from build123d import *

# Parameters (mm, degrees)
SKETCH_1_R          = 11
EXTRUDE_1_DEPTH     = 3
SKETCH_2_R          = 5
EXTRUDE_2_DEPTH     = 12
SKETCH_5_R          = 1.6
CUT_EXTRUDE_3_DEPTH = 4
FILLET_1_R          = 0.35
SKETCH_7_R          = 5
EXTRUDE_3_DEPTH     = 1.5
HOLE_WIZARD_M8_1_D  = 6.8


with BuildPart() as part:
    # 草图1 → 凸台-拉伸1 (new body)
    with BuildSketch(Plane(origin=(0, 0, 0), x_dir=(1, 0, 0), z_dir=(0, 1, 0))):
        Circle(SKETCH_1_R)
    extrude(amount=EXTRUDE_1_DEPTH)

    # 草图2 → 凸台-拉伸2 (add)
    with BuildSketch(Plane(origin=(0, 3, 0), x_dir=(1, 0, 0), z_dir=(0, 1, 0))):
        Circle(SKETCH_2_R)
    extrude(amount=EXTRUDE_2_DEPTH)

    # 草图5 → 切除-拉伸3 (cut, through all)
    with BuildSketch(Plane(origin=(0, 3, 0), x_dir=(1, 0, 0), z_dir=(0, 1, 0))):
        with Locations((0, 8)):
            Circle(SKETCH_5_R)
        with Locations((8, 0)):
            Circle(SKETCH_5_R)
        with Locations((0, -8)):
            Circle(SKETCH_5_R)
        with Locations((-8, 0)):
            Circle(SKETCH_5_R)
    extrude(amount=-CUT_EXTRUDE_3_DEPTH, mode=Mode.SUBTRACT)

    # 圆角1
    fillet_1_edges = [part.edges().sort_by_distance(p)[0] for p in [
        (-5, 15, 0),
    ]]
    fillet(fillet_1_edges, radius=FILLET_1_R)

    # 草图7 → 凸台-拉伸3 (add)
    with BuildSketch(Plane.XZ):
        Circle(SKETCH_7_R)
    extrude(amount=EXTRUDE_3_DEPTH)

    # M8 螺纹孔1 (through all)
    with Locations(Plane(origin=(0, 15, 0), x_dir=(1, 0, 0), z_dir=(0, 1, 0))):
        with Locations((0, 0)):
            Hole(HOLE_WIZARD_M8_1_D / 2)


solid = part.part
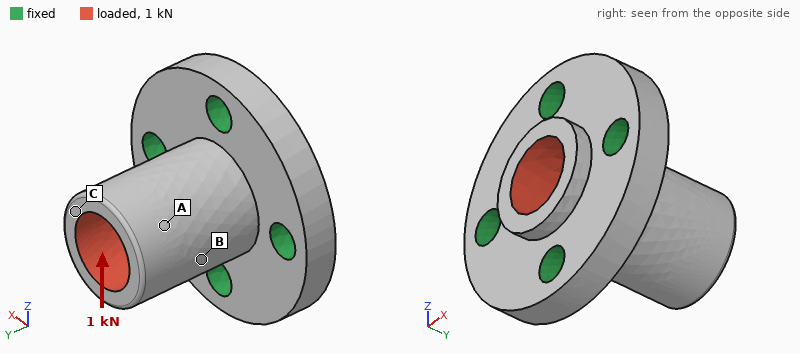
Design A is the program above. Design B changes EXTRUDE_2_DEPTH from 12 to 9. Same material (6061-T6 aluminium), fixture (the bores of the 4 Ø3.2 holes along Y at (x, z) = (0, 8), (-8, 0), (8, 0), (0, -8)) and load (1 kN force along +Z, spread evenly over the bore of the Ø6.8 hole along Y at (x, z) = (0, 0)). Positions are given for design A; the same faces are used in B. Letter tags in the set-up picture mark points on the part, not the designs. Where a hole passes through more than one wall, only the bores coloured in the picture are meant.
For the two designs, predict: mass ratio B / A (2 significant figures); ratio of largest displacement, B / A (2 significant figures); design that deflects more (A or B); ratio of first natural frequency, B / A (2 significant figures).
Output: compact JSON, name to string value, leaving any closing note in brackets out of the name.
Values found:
{"mass ratio B / A": "0.92", "ratio of largest displacement, B / A": "0.58", "design that deflects more": "A", "ratio of first natural frequency, B / A": "1.4"}
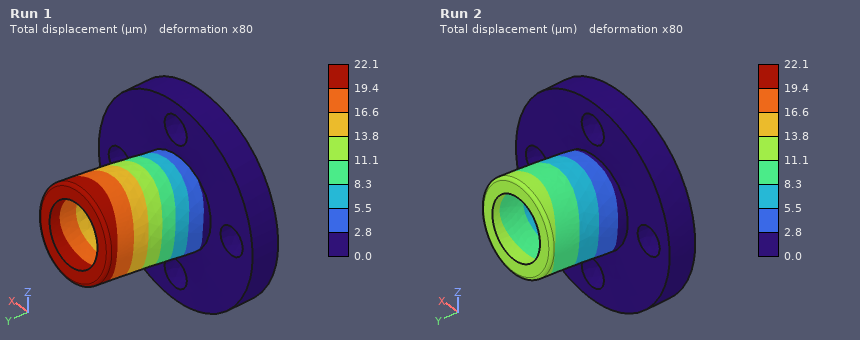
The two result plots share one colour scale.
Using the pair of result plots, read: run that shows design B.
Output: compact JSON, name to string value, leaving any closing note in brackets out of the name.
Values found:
{"run that shows design B": "Run 2"}
